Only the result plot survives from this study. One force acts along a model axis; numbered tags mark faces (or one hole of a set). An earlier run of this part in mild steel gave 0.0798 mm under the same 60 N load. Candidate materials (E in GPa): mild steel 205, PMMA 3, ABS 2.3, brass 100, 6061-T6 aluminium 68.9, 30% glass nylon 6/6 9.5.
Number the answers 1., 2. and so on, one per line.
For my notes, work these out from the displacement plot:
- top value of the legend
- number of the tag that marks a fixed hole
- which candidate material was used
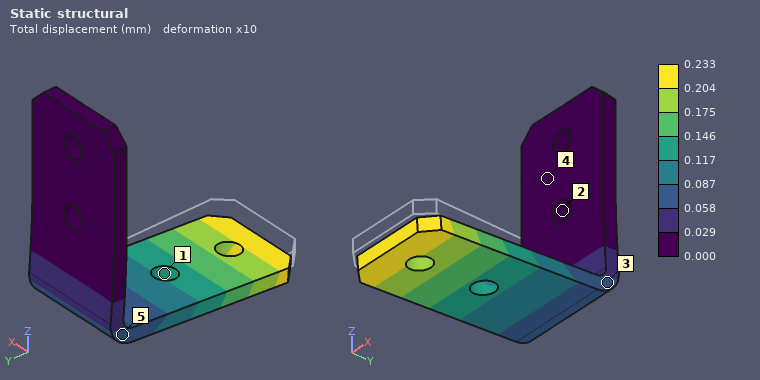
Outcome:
1. 0.233 mm
2. 2
3. 6061-T6 aluminium
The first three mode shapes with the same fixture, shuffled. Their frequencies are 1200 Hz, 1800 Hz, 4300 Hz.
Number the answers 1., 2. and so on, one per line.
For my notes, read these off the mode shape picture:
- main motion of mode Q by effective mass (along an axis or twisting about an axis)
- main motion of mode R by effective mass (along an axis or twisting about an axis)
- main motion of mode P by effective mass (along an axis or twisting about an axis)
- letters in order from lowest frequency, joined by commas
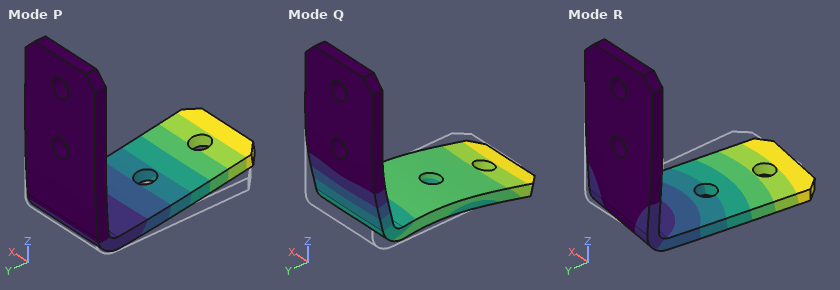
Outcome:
1. along Y
2. along X
3. along Z
4. P, R, Q
